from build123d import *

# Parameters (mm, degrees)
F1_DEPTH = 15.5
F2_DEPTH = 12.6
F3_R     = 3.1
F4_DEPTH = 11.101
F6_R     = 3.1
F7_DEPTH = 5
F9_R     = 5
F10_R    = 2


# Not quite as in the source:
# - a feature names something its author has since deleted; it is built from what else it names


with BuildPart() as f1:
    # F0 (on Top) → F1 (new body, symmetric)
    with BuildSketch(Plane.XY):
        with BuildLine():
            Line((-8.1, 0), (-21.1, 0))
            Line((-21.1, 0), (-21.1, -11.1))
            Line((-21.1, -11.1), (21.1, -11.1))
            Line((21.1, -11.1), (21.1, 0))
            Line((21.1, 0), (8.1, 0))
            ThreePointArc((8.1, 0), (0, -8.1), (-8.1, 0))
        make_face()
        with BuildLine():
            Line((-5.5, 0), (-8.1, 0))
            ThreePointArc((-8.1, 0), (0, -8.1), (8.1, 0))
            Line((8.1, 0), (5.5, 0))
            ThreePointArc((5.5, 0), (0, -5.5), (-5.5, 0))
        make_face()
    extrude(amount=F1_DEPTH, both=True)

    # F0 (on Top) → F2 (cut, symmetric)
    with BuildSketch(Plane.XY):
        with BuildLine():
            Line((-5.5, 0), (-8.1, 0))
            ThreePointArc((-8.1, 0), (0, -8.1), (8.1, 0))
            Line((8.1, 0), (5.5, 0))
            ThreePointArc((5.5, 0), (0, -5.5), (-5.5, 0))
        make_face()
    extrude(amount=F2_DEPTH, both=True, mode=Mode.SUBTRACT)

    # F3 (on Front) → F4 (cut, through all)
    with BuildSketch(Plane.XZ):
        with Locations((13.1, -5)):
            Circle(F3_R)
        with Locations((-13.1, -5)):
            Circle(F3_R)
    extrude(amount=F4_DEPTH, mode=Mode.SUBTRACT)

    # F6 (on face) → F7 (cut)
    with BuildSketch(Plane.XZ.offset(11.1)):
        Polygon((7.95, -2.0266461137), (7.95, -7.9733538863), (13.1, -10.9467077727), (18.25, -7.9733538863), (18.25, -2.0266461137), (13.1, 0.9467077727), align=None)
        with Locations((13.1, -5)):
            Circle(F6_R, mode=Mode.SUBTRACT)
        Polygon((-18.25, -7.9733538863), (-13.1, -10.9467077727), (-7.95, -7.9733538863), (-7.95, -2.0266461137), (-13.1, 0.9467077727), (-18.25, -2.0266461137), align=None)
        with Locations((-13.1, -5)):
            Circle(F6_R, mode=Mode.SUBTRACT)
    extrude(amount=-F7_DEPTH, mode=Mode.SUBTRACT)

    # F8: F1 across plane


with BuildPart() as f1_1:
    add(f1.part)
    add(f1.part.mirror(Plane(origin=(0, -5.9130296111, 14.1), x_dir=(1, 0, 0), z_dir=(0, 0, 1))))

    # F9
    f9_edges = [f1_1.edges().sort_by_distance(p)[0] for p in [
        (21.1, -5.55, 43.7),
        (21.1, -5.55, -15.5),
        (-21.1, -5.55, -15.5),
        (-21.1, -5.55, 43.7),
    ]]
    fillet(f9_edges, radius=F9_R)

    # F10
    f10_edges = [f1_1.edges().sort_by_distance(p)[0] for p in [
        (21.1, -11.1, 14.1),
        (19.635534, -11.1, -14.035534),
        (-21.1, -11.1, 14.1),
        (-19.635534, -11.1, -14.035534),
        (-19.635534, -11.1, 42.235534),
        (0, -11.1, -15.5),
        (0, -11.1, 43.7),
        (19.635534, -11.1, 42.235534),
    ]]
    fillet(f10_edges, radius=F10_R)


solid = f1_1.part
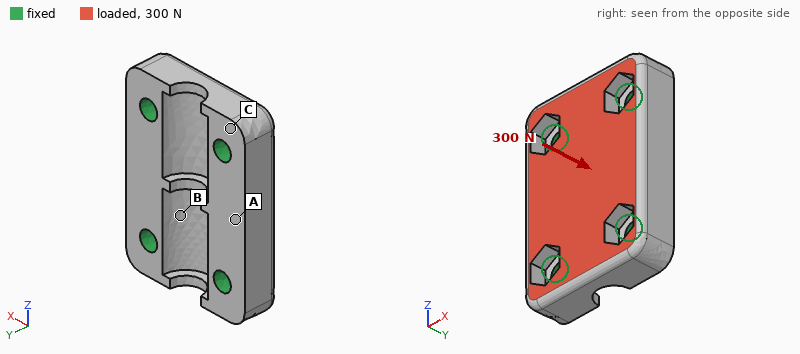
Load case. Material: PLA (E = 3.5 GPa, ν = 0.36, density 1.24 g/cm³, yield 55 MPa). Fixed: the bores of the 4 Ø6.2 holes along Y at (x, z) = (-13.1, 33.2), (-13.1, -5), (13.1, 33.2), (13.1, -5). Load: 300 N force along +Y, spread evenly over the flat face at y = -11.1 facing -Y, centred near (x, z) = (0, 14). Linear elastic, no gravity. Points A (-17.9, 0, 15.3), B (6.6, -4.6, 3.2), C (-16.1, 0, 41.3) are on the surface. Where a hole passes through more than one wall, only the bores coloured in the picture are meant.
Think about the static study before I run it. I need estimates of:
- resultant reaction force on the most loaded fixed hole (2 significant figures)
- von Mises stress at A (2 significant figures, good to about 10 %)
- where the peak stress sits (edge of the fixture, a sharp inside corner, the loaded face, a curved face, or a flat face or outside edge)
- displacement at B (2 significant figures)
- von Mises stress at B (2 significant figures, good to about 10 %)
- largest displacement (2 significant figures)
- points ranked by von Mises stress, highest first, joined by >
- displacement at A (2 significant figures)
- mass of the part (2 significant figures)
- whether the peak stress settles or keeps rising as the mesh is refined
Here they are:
86 N
0.63 MPa
edge of the fixture
5.6 µm
1.0 MPa
11 µm
B > A > C
5.7 µm
24 g
keeps rising
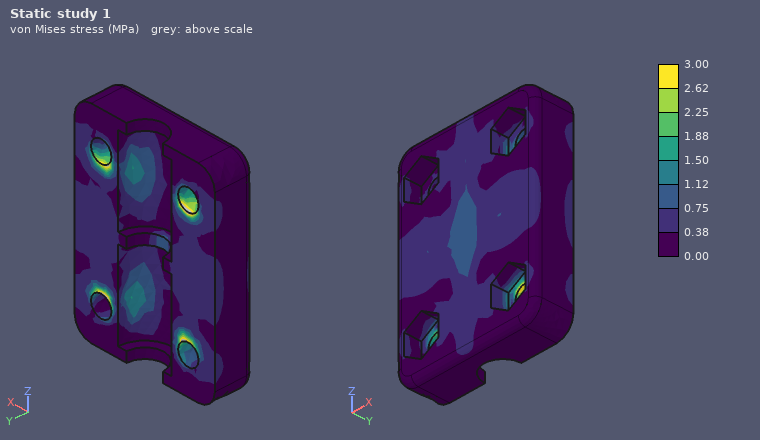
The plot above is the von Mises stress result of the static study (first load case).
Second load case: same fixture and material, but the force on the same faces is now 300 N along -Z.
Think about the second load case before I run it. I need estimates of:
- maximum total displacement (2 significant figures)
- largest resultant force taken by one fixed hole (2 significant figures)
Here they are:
6.7 µm
80 N
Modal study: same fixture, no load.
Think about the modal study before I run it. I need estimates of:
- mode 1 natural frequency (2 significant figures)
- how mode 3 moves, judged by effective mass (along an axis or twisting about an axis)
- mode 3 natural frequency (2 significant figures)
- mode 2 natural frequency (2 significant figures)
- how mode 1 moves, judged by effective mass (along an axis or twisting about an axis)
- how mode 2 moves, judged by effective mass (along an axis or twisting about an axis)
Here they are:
7700 Hz
along X
9200 Hz
8400 Hz
along Y
twisting about Z
